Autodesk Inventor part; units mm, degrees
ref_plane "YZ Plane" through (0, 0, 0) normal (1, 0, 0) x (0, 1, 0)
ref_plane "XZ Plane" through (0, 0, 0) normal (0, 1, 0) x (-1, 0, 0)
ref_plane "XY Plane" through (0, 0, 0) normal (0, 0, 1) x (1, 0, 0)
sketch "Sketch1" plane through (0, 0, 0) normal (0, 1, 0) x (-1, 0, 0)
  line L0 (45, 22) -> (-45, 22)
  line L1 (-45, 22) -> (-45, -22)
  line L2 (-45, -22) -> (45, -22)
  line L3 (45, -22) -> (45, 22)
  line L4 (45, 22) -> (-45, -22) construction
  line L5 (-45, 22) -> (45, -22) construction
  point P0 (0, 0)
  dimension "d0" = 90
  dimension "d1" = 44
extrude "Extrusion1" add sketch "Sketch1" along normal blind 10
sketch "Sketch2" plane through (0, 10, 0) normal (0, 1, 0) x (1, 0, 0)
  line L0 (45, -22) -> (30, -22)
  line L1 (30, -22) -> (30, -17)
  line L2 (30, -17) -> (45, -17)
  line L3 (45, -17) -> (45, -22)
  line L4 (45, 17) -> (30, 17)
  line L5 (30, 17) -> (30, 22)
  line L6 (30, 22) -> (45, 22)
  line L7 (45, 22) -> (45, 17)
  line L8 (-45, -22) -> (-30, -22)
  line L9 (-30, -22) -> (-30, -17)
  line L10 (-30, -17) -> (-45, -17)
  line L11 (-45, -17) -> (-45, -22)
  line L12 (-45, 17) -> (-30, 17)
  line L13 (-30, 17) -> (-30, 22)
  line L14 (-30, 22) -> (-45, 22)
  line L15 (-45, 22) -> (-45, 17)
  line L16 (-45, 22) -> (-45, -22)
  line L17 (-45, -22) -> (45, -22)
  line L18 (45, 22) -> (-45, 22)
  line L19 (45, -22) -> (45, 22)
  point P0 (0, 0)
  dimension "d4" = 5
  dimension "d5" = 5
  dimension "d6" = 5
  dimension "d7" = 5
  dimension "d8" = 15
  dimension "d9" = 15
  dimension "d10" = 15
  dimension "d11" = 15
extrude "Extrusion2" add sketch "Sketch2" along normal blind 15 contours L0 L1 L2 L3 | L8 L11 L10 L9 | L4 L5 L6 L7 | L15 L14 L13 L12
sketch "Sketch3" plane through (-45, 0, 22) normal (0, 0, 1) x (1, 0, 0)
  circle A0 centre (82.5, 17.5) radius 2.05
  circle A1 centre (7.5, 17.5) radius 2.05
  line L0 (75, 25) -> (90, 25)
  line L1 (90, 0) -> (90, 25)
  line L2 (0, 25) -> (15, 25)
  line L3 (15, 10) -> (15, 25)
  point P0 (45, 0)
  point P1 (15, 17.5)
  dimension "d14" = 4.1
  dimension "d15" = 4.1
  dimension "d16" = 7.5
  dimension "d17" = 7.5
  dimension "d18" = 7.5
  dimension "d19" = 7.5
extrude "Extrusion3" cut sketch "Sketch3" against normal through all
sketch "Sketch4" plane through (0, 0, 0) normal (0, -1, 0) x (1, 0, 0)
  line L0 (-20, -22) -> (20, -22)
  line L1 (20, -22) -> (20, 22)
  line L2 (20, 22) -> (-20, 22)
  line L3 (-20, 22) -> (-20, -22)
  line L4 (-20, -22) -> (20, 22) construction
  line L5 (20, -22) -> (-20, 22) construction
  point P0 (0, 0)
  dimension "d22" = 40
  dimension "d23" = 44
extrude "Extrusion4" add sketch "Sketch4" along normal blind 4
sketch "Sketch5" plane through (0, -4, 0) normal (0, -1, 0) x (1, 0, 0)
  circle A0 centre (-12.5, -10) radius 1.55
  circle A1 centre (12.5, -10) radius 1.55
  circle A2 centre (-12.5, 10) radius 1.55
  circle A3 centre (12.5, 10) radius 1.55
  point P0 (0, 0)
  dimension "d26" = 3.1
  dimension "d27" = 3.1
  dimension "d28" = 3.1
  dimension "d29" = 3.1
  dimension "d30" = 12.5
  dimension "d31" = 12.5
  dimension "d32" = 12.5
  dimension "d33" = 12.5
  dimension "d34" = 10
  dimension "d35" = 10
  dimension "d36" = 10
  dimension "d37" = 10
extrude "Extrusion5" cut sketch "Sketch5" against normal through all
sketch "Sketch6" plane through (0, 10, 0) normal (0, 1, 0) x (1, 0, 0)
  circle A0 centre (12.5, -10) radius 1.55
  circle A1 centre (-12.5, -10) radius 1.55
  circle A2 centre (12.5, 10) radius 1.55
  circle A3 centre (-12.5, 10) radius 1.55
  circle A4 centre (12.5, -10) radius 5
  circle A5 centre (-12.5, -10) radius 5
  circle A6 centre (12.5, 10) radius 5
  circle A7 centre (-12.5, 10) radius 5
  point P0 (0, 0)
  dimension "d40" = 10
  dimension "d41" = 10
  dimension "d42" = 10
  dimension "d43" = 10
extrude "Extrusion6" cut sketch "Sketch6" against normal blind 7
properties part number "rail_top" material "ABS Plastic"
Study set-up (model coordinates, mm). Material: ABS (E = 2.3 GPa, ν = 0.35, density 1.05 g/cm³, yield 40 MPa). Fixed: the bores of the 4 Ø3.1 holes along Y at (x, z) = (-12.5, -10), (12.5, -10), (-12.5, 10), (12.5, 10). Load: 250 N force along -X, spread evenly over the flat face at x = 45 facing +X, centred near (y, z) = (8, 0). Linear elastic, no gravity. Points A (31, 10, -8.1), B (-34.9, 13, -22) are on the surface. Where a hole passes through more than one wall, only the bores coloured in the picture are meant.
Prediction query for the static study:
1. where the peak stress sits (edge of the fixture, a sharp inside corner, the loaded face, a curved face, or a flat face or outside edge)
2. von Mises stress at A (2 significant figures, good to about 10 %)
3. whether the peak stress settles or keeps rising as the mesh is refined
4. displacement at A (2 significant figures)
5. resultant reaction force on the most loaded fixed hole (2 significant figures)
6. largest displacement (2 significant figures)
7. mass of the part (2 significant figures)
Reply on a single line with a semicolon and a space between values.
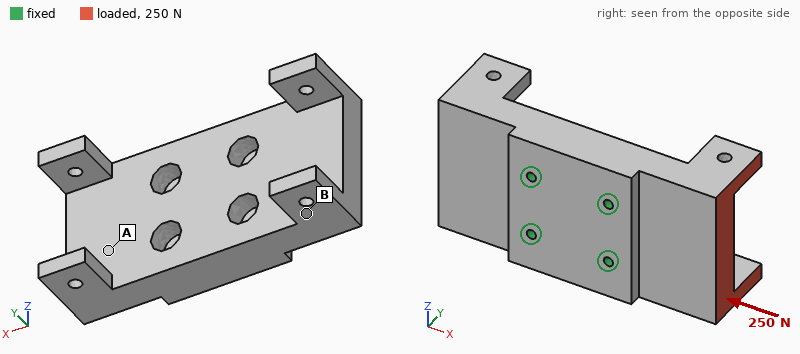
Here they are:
edge of the fixture; 1.2 MPa; keeps rising; 0.043 mm; 75 N; 0.13 mm; 51 g
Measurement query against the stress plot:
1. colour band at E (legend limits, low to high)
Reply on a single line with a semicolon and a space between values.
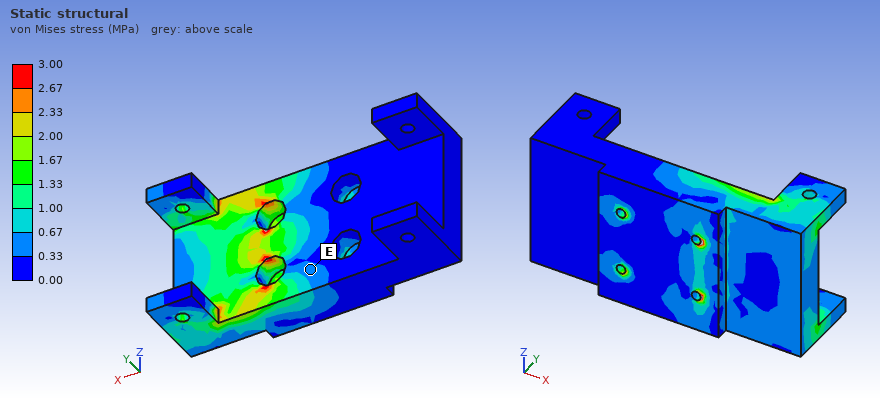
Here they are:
0.33 to 0.67 MPa
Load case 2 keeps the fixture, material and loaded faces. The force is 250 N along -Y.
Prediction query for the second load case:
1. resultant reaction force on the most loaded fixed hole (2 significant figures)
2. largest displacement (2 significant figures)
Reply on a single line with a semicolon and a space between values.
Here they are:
280 N; 0.56 mm
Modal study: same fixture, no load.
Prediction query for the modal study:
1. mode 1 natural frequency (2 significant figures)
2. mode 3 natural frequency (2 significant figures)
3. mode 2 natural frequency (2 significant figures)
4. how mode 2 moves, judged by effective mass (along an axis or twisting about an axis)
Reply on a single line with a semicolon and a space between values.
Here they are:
1500 Hz; 2200 Hz; 1600 Hz; along Y
